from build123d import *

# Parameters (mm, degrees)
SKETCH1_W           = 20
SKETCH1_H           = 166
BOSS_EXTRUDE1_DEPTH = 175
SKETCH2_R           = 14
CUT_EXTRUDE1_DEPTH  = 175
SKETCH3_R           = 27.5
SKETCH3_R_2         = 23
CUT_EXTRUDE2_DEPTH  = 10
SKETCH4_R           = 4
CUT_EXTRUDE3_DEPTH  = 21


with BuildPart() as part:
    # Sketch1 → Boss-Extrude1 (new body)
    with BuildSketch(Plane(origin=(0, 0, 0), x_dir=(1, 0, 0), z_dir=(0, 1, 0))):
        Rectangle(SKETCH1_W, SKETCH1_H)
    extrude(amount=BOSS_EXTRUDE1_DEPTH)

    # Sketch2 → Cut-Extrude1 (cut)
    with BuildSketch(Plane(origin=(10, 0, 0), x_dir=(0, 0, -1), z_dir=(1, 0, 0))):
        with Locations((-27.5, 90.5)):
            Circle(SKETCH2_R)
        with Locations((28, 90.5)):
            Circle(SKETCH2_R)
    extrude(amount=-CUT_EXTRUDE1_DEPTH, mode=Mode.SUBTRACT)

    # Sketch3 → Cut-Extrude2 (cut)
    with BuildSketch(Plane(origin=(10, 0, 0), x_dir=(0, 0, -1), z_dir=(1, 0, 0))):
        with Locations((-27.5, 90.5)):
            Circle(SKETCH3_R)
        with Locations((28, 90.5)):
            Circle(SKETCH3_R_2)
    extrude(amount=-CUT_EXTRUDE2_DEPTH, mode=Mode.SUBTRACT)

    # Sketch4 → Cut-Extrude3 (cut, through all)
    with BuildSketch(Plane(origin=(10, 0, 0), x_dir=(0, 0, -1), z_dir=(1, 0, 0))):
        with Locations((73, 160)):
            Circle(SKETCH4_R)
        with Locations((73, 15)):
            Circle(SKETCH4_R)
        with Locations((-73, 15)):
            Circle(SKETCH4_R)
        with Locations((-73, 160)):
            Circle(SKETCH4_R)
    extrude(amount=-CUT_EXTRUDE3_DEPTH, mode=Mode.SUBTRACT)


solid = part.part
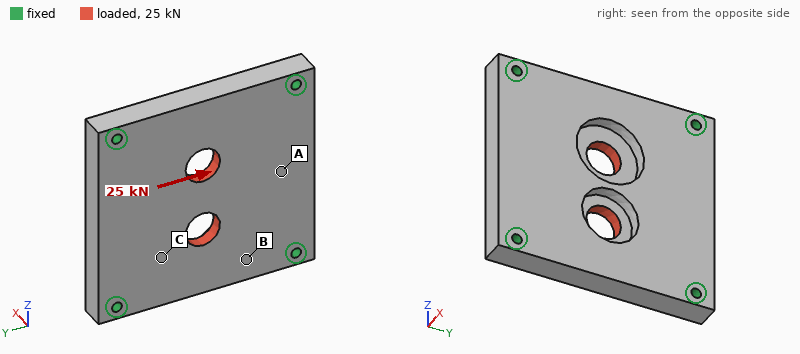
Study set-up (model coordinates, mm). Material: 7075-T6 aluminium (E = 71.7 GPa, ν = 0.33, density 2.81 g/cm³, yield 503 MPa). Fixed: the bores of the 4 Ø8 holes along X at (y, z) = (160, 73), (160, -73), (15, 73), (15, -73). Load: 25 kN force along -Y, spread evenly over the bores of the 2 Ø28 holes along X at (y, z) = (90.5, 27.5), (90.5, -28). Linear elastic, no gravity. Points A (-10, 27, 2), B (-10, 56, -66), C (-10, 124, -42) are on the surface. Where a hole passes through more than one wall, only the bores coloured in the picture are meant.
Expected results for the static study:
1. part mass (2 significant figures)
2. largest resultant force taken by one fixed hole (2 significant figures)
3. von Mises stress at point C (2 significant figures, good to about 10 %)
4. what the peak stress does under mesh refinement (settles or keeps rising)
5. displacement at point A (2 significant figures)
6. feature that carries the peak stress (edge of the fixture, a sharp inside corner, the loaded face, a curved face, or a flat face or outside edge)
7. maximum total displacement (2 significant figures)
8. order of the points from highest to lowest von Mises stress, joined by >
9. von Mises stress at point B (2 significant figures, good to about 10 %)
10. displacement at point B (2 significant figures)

1.5 kg
7.0 kN
12 MPa
keeps rising
12 µm
edge of the fixture
17 µm
C > B > A
7.5 MPa
5.3 µm
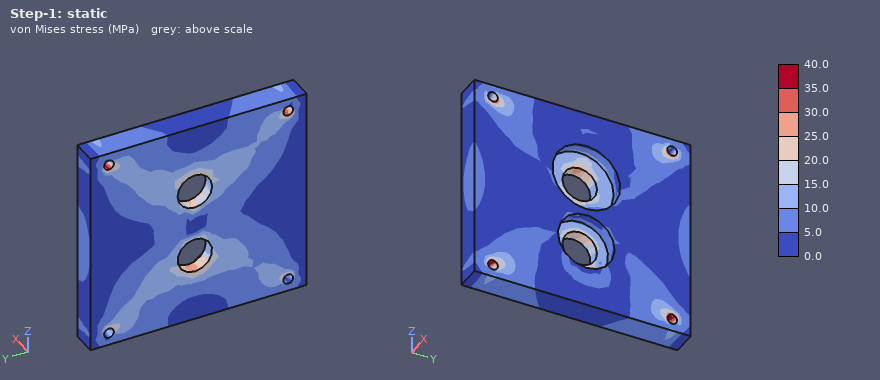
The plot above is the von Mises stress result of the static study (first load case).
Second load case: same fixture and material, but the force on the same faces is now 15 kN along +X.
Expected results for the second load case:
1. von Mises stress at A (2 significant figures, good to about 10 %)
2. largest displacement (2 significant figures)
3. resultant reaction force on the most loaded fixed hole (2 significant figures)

15 MPa
0.17 mm
4.5 kN
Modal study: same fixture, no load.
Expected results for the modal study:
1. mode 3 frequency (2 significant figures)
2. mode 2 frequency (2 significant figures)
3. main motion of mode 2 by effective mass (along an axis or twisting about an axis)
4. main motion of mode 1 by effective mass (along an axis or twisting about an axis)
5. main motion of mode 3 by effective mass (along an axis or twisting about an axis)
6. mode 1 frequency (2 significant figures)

4600 Hz
4300 Hz
twisting about Z
along X
twisting about Y
2700 Hz
